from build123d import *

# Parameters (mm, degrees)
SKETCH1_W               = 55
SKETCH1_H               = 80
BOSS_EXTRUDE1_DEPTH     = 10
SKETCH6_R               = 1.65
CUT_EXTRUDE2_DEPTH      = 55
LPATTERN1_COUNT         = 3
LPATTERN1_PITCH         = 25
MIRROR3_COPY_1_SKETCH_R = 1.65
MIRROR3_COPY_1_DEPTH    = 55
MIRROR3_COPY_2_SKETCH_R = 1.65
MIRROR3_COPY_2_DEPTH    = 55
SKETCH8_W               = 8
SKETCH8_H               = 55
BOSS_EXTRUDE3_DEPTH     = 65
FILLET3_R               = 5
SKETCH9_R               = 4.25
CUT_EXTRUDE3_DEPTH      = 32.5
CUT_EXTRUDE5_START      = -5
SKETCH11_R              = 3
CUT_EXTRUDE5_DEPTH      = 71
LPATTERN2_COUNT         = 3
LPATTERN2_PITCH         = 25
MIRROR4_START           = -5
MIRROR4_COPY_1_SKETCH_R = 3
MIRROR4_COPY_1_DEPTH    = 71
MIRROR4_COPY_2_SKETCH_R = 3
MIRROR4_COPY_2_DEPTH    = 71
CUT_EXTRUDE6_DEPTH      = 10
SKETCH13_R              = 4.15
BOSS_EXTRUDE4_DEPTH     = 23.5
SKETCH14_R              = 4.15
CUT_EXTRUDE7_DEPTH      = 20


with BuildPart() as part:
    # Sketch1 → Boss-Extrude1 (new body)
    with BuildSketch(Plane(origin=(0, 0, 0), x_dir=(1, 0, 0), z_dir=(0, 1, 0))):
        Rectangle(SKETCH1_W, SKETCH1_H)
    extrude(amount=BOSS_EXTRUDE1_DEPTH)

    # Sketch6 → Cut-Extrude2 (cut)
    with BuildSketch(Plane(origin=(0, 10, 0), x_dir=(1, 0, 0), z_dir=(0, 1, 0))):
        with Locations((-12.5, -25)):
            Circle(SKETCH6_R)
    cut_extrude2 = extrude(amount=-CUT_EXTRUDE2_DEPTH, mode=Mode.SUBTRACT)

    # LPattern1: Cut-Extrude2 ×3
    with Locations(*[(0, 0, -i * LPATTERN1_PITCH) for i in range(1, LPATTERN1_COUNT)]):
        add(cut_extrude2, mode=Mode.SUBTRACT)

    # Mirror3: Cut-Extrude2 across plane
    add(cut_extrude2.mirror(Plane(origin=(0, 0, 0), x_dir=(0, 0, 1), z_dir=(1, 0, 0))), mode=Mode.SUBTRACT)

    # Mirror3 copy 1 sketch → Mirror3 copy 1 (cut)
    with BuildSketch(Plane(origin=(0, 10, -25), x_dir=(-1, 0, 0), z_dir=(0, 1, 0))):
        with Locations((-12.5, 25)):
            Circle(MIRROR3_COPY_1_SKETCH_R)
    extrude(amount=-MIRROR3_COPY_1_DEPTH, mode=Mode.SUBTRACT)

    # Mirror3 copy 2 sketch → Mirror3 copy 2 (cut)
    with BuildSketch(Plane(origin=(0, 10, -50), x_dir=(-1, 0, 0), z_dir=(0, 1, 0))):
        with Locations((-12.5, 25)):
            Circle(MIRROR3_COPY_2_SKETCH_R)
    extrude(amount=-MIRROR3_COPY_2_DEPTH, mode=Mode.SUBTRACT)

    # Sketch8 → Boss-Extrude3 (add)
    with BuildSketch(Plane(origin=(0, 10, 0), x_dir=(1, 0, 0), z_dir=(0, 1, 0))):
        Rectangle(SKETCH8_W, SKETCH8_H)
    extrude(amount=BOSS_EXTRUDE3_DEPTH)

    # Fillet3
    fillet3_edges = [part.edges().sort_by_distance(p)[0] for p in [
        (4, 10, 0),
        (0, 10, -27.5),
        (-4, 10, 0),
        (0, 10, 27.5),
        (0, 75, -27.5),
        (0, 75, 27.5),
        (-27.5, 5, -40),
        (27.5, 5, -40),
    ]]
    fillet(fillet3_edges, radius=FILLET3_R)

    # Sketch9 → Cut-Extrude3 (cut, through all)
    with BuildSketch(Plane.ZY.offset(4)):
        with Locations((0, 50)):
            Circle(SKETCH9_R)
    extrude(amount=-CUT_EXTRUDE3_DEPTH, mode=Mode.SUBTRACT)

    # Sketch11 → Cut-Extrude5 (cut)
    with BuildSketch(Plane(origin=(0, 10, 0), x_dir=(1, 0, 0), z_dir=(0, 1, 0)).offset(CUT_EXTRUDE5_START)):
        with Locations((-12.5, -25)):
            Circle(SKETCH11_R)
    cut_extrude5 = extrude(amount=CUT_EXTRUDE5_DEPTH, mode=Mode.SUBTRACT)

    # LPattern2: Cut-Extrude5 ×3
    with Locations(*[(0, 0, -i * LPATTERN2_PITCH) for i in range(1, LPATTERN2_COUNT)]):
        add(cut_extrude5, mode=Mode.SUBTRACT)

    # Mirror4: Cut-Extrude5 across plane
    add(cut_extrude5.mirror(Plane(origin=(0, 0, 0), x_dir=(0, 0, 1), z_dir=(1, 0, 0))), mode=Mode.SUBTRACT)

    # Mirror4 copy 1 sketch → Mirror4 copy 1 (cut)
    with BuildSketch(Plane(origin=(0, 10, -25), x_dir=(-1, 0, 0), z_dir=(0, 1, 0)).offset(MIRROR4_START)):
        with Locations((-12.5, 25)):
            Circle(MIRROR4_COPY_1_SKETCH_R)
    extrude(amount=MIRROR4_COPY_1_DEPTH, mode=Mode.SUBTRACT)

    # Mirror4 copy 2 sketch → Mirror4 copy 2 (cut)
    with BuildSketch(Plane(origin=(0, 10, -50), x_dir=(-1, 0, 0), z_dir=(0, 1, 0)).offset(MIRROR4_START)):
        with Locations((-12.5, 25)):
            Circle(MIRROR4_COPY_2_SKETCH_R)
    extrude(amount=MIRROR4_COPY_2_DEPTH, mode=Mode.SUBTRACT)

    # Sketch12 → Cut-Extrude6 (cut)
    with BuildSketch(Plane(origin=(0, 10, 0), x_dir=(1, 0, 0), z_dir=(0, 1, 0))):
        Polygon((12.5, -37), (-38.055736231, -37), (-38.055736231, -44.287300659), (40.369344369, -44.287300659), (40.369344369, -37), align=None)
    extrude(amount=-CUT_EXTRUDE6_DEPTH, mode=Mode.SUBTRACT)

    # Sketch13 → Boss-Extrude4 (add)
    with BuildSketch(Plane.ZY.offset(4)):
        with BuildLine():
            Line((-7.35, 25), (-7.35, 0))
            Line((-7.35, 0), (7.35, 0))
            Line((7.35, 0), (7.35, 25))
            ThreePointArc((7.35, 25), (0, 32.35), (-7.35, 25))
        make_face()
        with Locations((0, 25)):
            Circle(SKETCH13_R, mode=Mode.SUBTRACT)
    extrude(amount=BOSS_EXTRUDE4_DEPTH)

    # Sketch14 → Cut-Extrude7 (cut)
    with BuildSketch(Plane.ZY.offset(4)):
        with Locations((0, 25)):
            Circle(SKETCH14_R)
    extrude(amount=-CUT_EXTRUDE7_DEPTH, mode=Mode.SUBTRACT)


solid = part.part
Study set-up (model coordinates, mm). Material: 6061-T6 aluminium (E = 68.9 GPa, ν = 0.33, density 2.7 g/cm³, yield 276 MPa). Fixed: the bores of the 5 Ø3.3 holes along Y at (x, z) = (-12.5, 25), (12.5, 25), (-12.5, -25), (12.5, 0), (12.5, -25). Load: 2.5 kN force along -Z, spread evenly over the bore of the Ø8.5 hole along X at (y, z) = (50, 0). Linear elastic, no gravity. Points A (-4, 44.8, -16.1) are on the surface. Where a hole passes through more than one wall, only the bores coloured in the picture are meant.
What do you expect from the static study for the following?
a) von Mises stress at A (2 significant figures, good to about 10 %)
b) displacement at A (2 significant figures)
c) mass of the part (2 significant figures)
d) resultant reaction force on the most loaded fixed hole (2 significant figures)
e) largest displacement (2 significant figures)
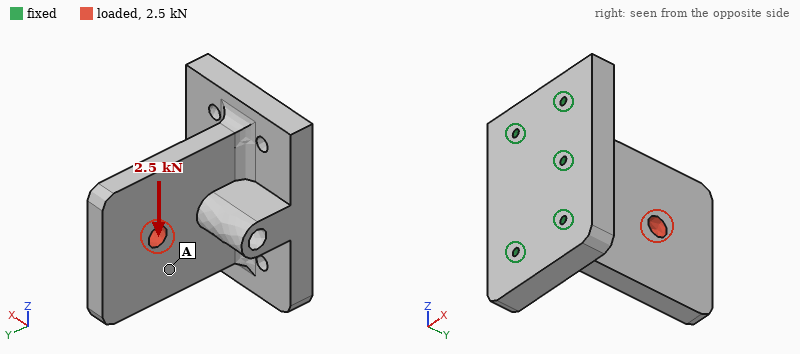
8.3 MPa
23 µm
200 g
1.4 kN
39 µm
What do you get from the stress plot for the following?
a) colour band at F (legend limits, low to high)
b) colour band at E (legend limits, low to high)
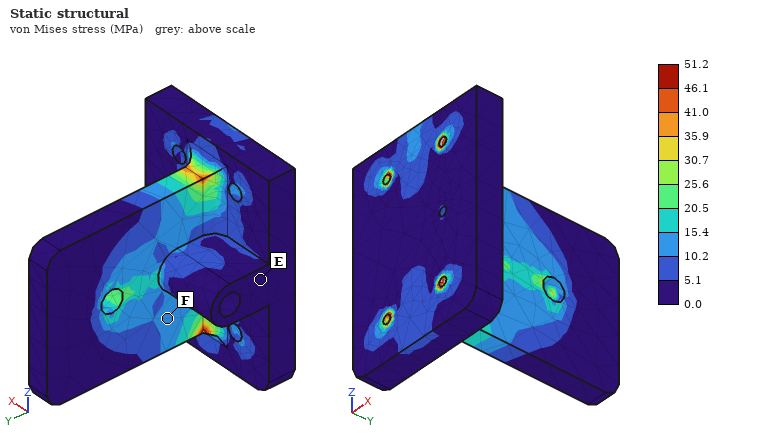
10.2 to 15.4 MPa
0.0 to 5.1 MPa
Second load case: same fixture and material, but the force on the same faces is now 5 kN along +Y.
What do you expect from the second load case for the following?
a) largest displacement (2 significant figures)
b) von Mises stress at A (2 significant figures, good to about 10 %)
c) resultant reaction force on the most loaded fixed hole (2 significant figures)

16 µm
8.6 MPa
1.3 kN
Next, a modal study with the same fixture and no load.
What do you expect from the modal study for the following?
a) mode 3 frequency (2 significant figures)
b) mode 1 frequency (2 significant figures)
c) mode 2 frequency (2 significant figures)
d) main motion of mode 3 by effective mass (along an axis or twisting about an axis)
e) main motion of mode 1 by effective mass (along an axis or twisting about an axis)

5900 Hz
2000 Hz
4200 Hz
along Z
along X
